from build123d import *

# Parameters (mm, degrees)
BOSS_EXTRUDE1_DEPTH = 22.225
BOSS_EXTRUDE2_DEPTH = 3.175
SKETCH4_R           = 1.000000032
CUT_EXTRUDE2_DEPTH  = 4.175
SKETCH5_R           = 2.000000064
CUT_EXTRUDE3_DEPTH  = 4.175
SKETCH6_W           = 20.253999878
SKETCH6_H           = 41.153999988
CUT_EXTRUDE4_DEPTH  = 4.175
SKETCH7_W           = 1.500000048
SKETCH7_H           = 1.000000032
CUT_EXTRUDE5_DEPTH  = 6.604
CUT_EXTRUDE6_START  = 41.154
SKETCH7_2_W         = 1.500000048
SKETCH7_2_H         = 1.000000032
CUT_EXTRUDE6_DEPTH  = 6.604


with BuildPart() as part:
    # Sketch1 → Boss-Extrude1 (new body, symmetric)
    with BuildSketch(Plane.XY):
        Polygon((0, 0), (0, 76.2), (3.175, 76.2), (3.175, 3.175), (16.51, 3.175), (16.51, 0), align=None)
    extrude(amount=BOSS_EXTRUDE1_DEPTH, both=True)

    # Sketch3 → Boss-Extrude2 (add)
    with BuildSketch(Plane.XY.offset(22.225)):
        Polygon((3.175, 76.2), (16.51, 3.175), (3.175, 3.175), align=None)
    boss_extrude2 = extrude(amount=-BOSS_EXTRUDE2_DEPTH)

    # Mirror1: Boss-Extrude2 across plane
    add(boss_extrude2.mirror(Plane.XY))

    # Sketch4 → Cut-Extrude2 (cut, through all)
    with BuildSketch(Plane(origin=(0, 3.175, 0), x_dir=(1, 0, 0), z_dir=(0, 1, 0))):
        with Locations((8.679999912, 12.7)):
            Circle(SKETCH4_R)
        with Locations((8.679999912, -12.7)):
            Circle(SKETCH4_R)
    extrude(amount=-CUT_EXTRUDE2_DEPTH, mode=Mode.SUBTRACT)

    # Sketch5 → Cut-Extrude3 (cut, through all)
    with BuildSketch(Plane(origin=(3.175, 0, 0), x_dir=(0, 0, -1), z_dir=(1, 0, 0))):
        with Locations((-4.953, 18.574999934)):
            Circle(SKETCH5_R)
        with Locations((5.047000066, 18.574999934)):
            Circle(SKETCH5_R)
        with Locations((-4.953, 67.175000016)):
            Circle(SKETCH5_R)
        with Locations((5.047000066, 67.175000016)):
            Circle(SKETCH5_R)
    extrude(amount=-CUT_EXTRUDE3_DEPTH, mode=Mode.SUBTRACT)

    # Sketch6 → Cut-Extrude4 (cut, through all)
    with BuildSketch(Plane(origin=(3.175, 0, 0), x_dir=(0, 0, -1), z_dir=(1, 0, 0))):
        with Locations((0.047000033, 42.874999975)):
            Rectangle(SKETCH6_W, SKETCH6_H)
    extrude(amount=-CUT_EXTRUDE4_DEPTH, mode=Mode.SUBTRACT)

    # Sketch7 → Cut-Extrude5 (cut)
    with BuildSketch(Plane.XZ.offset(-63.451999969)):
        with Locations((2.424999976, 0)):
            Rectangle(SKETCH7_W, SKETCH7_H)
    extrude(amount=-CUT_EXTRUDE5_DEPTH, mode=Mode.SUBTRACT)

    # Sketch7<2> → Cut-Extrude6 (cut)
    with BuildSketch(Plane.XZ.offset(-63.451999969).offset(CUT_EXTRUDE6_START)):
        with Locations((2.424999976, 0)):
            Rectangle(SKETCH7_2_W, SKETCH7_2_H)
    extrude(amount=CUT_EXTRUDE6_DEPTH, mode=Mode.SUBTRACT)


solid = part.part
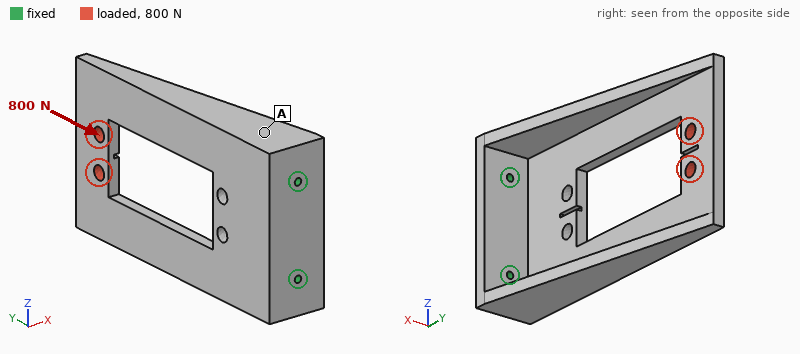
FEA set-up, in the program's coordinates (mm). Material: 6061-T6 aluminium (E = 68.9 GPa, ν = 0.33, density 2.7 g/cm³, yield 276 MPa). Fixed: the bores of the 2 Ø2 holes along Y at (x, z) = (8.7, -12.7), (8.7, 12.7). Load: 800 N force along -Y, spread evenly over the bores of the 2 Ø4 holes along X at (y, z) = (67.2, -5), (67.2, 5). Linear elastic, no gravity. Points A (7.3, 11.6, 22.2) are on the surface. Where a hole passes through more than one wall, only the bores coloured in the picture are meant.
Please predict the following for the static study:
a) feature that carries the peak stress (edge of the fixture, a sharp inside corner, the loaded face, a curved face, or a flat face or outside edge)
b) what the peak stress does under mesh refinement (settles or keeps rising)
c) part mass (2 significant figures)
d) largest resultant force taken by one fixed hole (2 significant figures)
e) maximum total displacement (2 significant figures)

edge of the fixture
keeps rising
35 g
400 N
0.27 mm
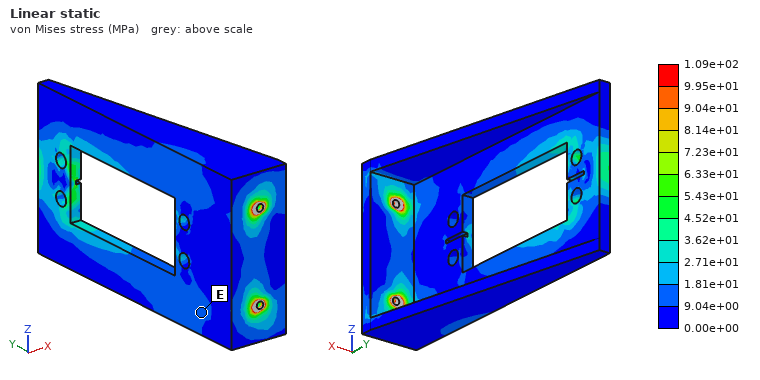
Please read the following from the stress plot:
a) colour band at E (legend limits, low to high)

9.04e+00 to 1.81e+01 MPa
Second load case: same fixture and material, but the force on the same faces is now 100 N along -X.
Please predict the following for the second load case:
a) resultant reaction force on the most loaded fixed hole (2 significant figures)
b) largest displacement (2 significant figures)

56 N
0.48 mm
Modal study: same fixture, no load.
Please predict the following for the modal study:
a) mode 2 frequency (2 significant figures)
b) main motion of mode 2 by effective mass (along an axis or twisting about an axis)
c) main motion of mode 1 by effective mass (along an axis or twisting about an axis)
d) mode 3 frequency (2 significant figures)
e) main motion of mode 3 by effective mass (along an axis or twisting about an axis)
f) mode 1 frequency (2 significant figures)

1500 Hz
along Z
along X
2800 Hz
along Z
810 Hz
